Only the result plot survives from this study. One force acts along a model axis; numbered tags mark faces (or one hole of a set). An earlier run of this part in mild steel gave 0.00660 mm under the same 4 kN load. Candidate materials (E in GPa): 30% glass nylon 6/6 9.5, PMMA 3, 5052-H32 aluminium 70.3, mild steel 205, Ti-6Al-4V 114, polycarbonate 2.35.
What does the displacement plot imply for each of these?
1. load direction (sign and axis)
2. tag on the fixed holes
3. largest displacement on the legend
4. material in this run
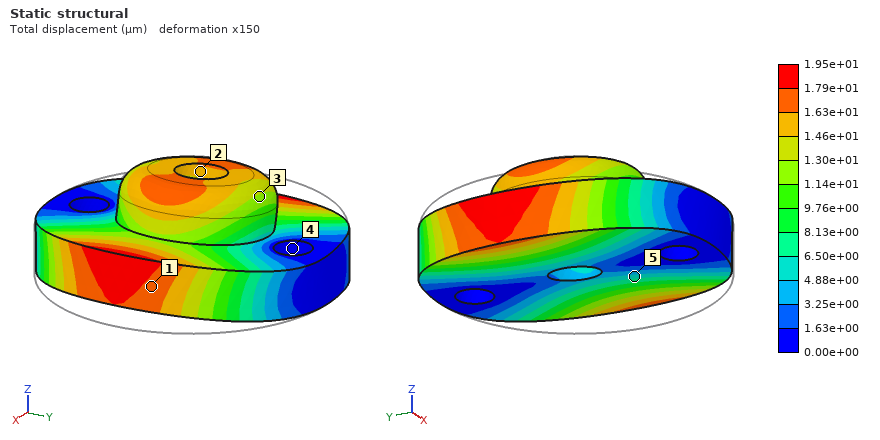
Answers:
-X
4
1.95e+01 µm
5052-H32 aluminium
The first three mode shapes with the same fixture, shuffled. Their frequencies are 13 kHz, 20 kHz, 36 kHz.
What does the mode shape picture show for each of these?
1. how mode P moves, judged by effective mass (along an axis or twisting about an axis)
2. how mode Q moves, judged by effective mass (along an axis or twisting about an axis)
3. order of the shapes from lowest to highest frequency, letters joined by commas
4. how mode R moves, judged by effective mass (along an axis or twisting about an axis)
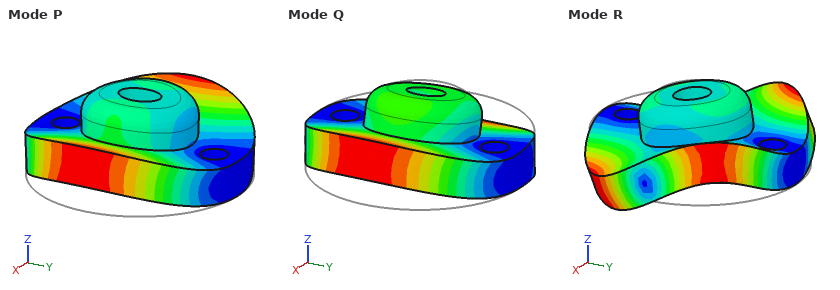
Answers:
along Z
twisting about Y
Q, P, R
twisting about X
